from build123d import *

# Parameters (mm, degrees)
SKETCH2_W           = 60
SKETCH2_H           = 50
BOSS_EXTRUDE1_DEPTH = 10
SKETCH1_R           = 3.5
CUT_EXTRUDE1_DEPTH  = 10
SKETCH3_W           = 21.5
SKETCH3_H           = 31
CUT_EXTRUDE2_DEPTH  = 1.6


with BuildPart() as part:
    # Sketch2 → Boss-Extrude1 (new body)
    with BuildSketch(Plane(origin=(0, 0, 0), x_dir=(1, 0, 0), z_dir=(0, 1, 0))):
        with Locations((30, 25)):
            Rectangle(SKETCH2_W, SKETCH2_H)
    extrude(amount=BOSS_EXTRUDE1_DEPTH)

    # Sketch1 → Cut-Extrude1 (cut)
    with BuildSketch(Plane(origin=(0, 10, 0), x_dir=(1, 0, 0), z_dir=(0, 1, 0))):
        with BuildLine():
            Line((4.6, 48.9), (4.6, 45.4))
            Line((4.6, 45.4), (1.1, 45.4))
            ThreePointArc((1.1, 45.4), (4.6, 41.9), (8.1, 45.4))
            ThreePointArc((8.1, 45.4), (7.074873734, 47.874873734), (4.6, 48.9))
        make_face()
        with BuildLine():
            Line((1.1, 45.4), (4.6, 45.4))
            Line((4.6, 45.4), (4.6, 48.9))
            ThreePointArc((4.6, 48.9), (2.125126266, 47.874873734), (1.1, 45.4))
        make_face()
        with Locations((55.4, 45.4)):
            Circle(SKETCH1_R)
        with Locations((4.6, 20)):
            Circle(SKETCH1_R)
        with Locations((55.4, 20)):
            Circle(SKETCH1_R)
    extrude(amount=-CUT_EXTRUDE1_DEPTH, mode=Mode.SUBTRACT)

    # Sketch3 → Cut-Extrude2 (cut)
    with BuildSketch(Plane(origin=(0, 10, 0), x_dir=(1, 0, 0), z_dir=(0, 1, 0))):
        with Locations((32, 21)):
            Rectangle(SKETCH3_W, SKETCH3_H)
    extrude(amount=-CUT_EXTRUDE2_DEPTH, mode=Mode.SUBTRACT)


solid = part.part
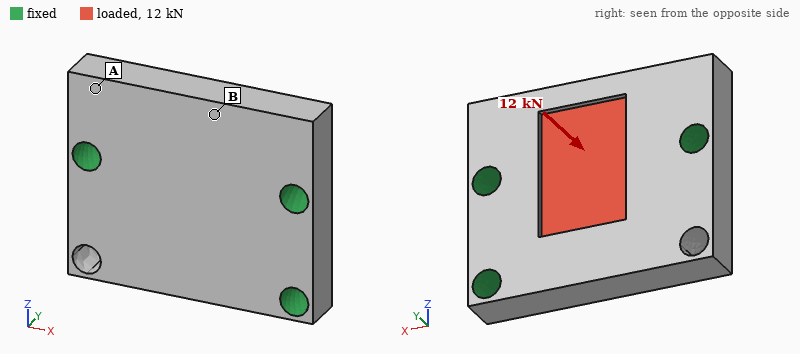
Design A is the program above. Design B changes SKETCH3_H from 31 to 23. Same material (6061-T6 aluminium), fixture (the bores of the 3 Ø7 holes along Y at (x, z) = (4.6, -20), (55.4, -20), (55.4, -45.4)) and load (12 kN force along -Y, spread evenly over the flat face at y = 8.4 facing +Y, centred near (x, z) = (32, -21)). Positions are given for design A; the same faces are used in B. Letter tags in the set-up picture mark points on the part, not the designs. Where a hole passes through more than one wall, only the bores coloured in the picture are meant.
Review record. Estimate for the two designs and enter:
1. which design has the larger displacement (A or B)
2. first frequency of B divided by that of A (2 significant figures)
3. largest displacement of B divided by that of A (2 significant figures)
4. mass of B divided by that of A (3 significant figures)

A
1.0
0.86
1.01
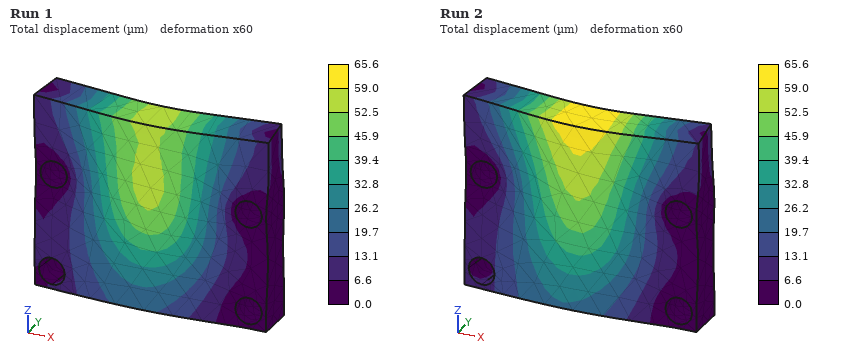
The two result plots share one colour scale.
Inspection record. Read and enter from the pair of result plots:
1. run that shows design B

Run 1
